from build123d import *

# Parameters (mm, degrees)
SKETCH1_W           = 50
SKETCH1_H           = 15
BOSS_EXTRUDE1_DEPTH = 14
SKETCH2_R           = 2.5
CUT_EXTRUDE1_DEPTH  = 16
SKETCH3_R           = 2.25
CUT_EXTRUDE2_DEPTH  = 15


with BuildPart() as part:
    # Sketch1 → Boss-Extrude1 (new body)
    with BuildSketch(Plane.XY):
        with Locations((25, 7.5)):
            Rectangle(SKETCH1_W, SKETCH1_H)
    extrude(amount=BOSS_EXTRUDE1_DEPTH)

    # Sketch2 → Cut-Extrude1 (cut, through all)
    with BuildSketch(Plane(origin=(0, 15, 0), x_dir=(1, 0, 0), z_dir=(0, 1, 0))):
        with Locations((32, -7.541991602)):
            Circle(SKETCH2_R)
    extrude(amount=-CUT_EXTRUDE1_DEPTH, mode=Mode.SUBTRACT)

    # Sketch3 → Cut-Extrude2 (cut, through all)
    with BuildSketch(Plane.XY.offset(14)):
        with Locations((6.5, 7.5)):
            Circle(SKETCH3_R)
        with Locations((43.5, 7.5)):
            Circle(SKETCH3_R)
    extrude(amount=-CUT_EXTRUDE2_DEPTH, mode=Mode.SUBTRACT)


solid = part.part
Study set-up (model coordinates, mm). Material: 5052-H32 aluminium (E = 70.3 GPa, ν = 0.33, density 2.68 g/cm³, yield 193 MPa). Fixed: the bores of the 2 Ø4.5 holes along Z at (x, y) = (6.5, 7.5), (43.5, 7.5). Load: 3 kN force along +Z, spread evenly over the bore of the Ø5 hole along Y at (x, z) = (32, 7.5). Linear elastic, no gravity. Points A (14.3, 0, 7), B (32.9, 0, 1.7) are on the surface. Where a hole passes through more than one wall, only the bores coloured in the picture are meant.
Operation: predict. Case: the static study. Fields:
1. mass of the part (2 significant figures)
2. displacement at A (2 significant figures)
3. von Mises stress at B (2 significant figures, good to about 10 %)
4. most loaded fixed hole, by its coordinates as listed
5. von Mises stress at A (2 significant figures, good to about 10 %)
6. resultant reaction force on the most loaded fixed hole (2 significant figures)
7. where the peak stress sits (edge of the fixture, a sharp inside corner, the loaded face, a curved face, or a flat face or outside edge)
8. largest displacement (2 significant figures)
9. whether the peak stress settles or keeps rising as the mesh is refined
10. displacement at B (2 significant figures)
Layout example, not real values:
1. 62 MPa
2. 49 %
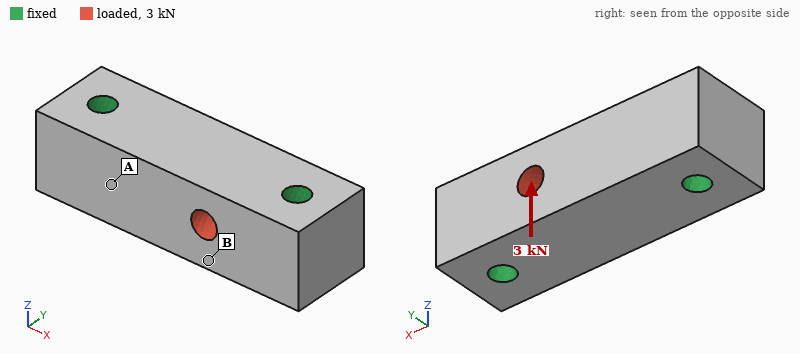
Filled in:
1. 26 g
2. 2.2 µm
3. 18 MPa
4. (43.5, 7.5)
5. 9.6 MPa
6. 2.2 kN
7. edge of the fixture
8. 8.2 µm
9. keeps rising
10. 6.4 µm
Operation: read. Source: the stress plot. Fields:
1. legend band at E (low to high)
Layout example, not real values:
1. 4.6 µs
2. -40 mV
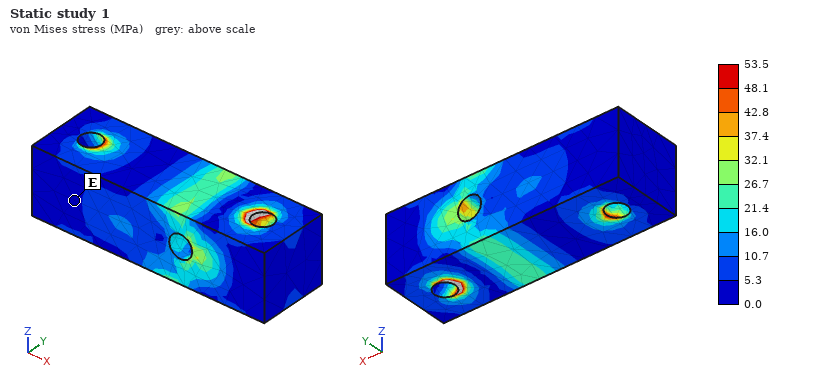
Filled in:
1. 0.0 to 5.3 MPa
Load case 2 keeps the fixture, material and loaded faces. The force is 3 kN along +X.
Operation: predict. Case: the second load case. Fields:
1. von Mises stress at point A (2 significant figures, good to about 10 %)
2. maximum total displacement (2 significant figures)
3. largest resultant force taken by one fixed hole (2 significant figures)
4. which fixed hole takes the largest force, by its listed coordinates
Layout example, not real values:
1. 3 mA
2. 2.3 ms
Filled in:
1. 3.9 MPa
2. 2.3 µm
3. 2.0 kN
4. (43.5, 7.5)
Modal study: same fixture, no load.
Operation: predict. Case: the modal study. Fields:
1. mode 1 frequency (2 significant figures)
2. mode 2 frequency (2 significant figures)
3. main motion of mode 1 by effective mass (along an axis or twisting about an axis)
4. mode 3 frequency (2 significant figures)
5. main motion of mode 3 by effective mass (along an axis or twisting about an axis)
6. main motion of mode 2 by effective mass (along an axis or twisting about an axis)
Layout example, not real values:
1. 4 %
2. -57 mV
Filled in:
1. 28 kHz
2. 31 kHz
3. along Y
4. 38 kHz
5. twisting about X
6. along Z
